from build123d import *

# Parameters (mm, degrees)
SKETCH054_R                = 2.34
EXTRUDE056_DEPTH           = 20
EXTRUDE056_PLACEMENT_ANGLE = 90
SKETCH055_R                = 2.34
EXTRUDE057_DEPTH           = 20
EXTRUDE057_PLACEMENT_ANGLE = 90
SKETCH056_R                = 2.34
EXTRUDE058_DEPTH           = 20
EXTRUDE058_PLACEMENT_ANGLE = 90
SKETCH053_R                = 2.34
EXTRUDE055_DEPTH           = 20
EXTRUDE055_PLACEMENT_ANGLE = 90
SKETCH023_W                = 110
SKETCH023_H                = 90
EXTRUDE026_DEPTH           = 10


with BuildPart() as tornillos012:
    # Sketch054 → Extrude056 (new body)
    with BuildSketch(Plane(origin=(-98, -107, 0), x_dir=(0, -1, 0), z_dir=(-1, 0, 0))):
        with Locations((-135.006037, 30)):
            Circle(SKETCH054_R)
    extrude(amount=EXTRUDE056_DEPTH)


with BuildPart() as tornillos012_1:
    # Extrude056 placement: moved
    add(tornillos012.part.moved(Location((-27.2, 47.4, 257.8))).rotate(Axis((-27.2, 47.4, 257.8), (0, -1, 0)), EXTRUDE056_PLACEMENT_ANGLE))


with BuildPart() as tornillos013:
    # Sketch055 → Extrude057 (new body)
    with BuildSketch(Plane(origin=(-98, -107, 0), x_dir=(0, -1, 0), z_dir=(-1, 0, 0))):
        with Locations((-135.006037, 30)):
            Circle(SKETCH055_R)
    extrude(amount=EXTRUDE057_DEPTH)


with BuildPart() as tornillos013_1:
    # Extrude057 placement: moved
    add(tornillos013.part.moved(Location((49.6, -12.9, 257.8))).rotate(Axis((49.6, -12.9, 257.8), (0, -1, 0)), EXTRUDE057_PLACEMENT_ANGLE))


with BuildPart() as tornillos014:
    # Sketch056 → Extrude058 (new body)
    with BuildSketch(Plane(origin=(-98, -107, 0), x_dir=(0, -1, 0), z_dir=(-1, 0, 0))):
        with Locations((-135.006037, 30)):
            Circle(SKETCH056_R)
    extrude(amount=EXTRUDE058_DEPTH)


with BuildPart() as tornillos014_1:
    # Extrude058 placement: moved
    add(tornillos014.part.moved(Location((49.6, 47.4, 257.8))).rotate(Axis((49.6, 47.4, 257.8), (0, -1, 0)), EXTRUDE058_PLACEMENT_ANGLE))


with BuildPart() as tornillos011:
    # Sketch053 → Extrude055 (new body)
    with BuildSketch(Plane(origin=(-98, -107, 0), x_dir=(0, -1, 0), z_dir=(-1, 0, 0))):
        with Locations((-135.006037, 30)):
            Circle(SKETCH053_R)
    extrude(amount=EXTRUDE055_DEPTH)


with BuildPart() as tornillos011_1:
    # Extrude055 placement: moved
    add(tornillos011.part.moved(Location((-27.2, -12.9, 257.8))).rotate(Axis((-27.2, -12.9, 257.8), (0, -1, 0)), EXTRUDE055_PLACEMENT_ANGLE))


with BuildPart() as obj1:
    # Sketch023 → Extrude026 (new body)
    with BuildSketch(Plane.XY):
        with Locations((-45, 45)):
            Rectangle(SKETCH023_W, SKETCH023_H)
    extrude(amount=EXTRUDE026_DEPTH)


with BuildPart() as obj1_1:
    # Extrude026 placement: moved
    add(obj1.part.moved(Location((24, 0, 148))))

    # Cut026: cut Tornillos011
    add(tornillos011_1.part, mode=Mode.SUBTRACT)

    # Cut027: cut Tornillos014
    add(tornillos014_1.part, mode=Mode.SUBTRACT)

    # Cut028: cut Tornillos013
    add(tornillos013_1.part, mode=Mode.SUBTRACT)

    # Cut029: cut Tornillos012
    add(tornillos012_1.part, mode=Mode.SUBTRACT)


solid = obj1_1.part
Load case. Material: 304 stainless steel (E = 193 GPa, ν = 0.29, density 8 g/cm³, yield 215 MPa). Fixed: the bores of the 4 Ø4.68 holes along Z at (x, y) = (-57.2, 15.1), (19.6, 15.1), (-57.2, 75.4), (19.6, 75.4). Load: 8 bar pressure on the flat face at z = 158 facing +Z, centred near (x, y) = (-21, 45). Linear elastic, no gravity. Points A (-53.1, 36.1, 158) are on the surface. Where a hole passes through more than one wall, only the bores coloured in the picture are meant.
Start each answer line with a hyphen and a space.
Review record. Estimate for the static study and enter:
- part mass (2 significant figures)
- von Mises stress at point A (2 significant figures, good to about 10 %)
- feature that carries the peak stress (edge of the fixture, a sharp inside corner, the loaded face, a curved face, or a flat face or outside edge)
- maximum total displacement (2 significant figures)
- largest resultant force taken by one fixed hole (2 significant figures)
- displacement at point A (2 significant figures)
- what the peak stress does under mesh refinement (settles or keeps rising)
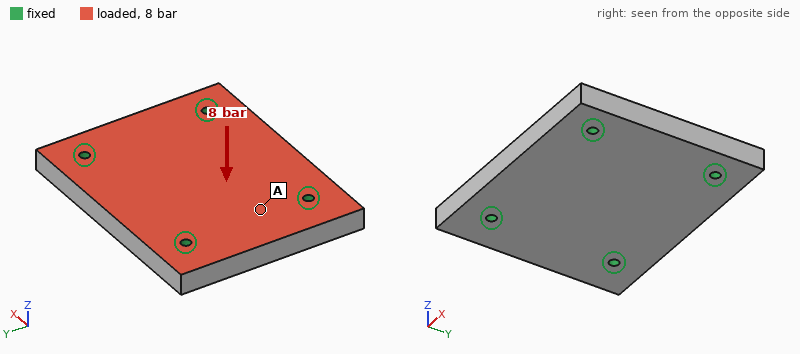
- 790 g
- 9.7 MPa
- edge of the fixture
- 9.5 µm
- 2.1 kN
- 4.3 µm
- keeps rising
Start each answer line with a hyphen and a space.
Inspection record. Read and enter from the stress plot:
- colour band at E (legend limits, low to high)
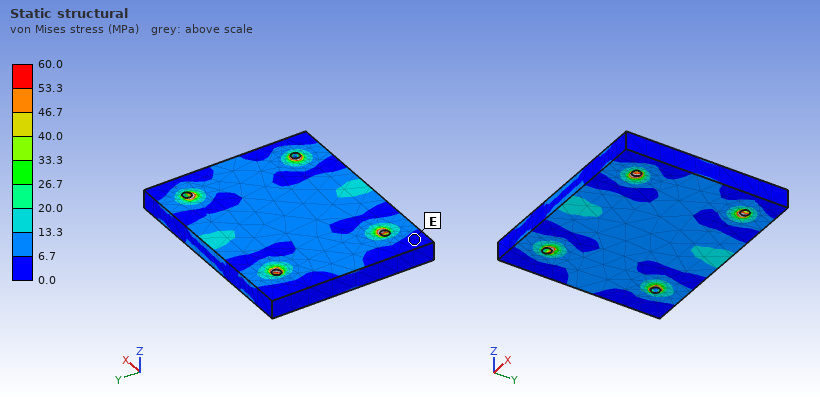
- 0.0 to 6.7 MPa
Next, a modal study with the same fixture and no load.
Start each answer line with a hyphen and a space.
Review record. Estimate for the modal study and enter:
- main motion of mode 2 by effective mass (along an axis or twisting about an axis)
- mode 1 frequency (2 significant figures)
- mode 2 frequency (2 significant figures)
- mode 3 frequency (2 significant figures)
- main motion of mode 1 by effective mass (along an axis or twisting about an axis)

- twisting about X
- 5900 Hz
- 7900 Hz
- 9100 Hz
- along Z
